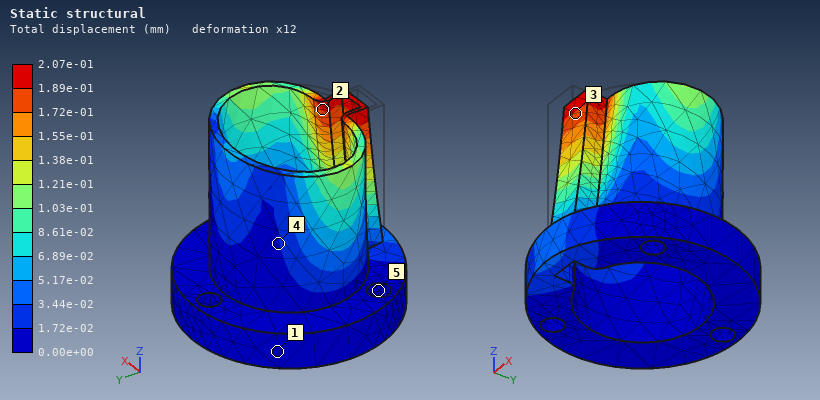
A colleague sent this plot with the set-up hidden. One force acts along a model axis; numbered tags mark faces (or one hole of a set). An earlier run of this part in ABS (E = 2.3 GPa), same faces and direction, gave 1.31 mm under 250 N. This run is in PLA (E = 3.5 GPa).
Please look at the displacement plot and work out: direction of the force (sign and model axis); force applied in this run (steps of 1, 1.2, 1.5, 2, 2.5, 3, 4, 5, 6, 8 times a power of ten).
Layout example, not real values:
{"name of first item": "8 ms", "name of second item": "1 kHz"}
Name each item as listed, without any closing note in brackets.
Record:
{"direction of the force": "+Y", "force applied in this run": "60 N"}
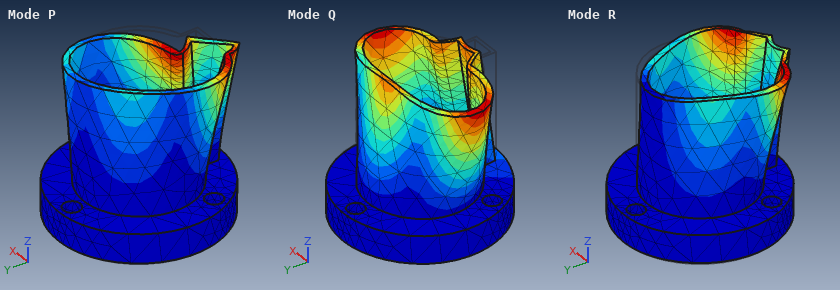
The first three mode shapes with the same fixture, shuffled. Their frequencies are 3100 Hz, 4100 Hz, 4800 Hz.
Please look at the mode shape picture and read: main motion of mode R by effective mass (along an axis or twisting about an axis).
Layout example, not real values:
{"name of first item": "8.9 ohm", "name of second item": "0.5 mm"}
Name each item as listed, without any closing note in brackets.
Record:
{"main motion of mode R by effective mass": "along Y"}
